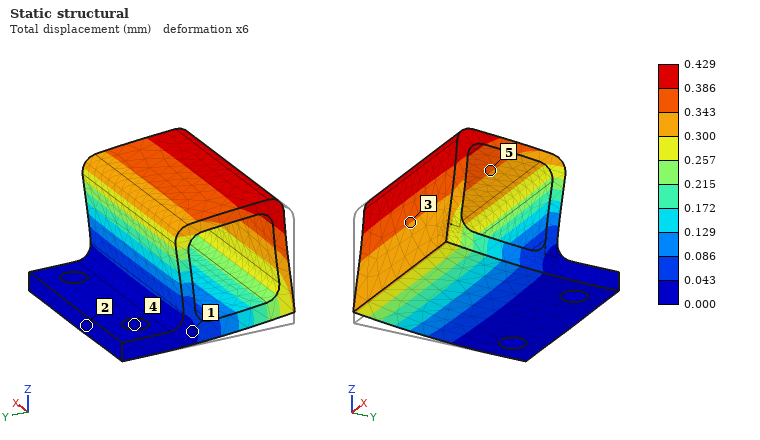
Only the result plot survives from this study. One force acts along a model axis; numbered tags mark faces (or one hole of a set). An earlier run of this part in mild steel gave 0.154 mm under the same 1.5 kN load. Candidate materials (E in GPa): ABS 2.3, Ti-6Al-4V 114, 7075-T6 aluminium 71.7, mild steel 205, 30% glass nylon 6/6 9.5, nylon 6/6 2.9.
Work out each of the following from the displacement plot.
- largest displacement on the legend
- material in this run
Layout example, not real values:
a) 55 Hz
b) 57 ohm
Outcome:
a) 0.429 mm
b) 7075-T6 aluminium
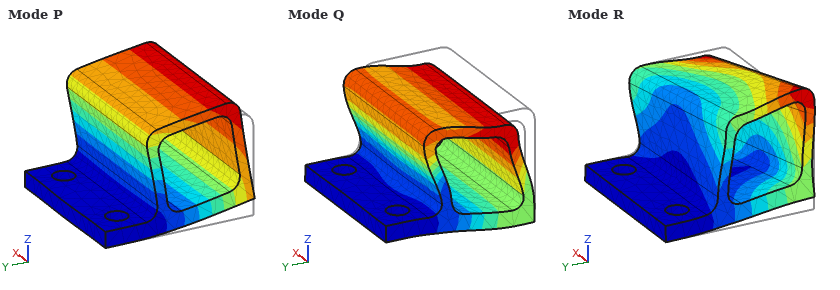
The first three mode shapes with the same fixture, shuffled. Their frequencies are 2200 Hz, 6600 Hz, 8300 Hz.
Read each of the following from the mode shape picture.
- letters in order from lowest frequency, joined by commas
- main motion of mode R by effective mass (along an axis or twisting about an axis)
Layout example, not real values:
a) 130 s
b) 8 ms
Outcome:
a) P, R, Q
b) along X
